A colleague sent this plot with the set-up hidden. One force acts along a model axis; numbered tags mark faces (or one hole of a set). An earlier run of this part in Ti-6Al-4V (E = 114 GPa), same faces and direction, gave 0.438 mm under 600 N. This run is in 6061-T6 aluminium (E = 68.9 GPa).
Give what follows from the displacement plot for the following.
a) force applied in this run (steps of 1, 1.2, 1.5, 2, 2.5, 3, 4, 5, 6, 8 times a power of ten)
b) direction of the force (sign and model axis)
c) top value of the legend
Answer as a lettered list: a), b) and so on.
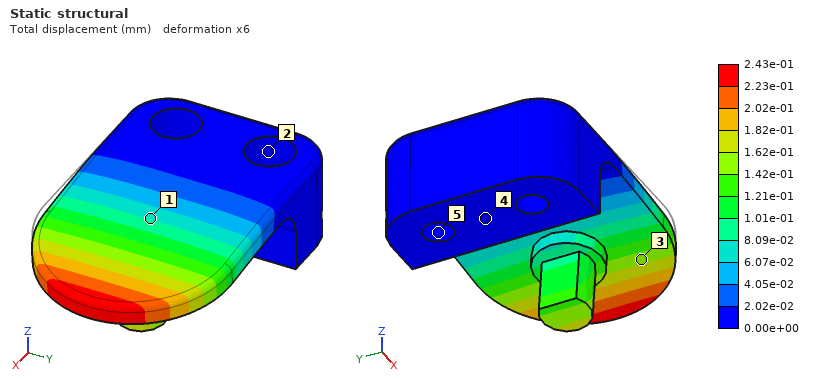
a) 200 N
b) -Z
c) 2.43e-01 mm
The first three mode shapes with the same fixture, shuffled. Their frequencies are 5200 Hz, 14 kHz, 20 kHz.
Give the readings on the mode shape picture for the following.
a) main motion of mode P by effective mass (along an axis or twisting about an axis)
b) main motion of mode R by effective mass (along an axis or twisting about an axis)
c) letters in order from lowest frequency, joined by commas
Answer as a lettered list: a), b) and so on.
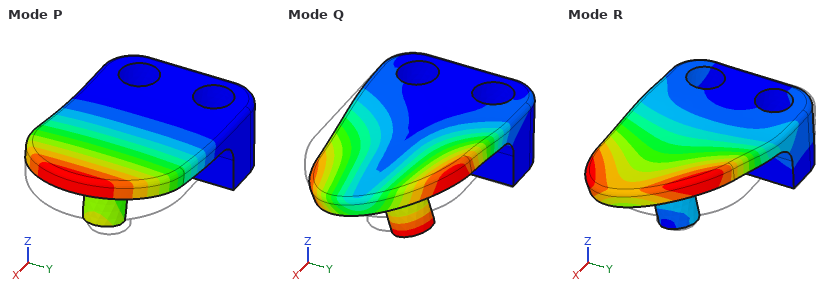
a) along Z
b) along Y
c) P, Q, R
